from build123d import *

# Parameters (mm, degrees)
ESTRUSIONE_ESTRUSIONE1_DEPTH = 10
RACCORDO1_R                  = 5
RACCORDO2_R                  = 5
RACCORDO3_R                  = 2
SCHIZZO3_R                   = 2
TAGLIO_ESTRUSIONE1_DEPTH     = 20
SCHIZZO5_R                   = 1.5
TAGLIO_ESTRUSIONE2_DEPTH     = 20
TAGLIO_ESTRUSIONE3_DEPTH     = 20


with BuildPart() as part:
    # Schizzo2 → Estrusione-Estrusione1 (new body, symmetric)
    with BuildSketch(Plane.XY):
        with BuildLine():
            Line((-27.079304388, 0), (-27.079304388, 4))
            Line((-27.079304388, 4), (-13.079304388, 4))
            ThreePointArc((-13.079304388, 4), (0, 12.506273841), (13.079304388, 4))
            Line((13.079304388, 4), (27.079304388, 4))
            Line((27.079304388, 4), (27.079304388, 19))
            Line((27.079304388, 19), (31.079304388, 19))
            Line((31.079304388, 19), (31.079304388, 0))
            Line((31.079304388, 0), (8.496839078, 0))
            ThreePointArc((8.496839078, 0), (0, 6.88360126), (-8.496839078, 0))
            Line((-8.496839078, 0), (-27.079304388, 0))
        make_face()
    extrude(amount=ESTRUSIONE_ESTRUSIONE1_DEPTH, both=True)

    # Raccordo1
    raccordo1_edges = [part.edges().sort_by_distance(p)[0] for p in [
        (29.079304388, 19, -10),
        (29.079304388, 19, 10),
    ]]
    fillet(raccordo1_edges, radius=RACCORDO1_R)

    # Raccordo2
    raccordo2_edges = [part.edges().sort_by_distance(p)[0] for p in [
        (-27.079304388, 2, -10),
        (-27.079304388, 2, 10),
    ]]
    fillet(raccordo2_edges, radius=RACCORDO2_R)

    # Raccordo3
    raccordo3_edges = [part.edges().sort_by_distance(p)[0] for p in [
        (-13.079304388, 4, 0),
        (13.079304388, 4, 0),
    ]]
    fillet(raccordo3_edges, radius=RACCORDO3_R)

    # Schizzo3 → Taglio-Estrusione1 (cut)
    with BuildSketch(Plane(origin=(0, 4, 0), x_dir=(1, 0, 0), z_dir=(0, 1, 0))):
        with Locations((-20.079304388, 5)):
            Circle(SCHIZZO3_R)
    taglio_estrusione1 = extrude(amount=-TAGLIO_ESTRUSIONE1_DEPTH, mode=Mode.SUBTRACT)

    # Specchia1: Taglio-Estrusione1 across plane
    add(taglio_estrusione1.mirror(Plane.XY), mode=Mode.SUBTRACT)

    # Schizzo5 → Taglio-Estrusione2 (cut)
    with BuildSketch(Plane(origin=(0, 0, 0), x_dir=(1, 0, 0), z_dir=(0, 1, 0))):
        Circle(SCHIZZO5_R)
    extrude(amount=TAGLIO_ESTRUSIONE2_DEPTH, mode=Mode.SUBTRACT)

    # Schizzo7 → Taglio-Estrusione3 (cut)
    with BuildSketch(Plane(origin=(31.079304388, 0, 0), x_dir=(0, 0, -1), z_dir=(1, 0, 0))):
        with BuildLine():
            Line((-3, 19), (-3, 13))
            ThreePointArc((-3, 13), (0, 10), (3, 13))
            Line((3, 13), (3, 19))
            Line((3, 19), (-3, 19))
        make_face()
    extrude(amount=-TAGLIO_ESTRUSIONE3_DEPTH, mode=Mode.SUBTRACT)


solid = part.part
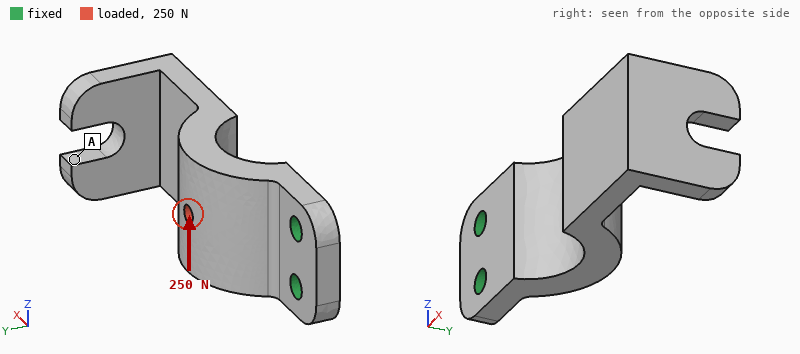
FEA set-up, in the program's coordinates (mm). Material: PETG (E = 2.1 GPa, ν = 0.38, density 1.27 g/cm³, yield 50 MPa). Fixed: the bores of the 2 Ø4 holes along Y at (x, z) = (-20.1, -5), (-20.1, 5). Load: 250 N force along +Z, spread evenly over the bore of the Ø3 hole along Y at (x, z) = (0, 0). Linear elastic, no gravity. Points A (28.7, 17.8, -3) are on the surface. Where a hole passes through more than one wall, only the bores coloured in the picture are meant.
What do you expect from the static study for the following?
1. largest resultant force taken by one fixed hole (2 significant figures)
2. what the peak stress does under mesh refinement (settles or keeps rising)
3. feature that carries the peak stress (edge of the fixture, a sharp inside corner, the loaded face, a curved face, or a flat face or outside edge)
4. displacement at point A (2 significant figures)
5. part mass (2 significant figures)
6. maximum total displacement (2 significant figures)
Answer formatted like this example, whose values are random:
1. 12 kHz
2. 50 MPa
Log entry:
1. 430 N
2. keeps rising
3. edge of the fixture
4. 0.68 mm
5. 8.8 g
6. 0.71 mm
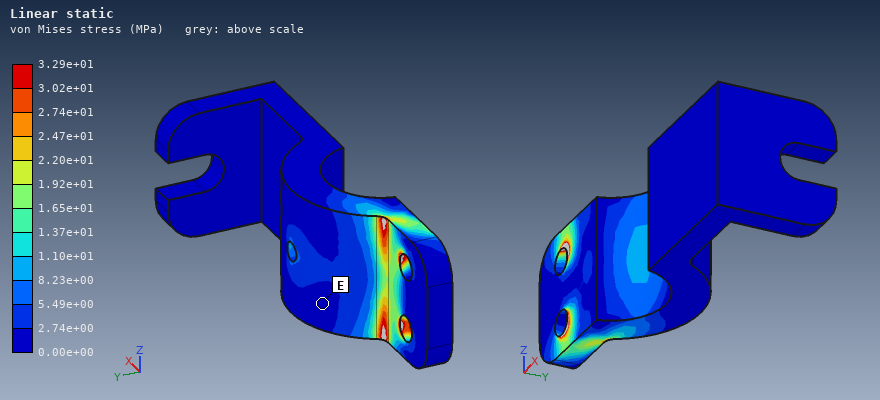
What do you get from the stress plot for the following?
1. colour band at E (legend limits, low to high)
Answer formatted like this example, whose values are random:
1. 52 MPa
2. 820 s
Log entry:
1. 0.00e+00 to 2.74e+00 MPa
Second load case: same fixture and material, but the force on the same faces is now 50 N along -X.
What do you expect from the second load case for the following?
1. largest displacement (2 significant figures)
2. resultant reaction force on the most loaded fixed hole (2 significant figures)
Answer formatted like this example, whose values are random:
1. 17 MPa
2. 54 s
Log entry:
1. 0.68 mm
2. 26 N
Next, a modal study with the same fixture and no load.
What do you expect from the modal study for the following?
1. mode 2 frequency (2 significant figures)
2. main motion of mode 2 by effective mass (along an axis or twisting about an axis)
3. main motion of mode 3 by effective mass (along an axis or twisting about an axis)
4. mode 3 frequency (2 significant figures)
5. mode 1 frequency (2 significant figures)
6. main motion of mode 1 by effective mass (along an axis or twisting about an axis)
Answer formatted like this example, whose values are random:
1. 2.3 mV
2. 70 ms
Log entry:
1. 750 Hz
2. along Z
3. twisting about X
4. 1200 Hz
5. 280 Hz
6. along Y
